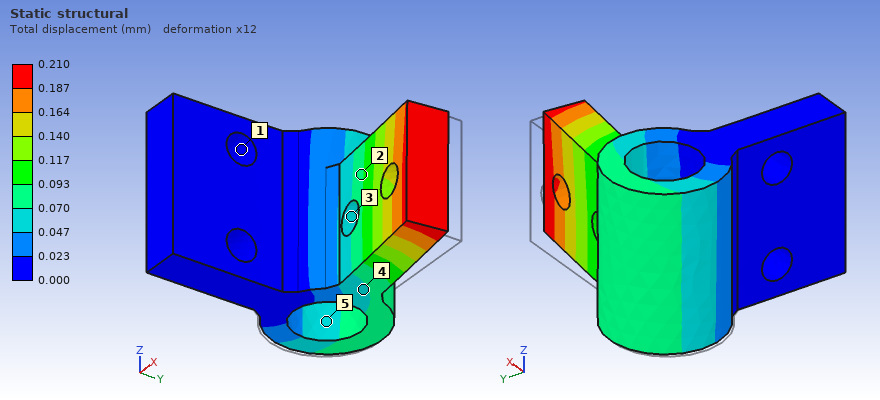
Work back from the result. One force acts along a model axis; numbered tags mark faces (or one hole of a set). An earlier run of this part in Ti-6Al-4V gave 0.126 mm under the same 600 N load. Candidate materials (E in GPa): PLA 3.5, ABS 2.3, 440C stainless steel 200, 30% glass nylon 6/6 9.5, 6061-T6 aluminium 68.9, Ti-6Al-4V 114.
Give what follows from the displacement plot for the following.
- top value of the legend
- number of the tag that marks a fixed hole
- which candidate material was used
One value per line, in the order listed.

0.210 mm
1
6061-T6 aluminium
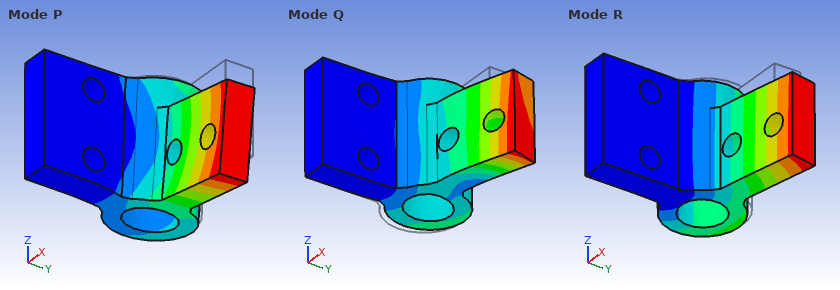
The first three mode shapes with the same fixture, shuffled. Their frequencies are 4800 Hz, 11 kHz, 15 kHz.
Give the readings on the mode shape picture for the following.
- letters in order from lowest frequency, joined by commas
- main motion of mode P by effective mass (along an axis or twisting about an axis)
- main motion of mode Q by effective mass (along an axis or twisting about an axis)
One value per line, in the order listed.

R, P, Q
along Z
along X
